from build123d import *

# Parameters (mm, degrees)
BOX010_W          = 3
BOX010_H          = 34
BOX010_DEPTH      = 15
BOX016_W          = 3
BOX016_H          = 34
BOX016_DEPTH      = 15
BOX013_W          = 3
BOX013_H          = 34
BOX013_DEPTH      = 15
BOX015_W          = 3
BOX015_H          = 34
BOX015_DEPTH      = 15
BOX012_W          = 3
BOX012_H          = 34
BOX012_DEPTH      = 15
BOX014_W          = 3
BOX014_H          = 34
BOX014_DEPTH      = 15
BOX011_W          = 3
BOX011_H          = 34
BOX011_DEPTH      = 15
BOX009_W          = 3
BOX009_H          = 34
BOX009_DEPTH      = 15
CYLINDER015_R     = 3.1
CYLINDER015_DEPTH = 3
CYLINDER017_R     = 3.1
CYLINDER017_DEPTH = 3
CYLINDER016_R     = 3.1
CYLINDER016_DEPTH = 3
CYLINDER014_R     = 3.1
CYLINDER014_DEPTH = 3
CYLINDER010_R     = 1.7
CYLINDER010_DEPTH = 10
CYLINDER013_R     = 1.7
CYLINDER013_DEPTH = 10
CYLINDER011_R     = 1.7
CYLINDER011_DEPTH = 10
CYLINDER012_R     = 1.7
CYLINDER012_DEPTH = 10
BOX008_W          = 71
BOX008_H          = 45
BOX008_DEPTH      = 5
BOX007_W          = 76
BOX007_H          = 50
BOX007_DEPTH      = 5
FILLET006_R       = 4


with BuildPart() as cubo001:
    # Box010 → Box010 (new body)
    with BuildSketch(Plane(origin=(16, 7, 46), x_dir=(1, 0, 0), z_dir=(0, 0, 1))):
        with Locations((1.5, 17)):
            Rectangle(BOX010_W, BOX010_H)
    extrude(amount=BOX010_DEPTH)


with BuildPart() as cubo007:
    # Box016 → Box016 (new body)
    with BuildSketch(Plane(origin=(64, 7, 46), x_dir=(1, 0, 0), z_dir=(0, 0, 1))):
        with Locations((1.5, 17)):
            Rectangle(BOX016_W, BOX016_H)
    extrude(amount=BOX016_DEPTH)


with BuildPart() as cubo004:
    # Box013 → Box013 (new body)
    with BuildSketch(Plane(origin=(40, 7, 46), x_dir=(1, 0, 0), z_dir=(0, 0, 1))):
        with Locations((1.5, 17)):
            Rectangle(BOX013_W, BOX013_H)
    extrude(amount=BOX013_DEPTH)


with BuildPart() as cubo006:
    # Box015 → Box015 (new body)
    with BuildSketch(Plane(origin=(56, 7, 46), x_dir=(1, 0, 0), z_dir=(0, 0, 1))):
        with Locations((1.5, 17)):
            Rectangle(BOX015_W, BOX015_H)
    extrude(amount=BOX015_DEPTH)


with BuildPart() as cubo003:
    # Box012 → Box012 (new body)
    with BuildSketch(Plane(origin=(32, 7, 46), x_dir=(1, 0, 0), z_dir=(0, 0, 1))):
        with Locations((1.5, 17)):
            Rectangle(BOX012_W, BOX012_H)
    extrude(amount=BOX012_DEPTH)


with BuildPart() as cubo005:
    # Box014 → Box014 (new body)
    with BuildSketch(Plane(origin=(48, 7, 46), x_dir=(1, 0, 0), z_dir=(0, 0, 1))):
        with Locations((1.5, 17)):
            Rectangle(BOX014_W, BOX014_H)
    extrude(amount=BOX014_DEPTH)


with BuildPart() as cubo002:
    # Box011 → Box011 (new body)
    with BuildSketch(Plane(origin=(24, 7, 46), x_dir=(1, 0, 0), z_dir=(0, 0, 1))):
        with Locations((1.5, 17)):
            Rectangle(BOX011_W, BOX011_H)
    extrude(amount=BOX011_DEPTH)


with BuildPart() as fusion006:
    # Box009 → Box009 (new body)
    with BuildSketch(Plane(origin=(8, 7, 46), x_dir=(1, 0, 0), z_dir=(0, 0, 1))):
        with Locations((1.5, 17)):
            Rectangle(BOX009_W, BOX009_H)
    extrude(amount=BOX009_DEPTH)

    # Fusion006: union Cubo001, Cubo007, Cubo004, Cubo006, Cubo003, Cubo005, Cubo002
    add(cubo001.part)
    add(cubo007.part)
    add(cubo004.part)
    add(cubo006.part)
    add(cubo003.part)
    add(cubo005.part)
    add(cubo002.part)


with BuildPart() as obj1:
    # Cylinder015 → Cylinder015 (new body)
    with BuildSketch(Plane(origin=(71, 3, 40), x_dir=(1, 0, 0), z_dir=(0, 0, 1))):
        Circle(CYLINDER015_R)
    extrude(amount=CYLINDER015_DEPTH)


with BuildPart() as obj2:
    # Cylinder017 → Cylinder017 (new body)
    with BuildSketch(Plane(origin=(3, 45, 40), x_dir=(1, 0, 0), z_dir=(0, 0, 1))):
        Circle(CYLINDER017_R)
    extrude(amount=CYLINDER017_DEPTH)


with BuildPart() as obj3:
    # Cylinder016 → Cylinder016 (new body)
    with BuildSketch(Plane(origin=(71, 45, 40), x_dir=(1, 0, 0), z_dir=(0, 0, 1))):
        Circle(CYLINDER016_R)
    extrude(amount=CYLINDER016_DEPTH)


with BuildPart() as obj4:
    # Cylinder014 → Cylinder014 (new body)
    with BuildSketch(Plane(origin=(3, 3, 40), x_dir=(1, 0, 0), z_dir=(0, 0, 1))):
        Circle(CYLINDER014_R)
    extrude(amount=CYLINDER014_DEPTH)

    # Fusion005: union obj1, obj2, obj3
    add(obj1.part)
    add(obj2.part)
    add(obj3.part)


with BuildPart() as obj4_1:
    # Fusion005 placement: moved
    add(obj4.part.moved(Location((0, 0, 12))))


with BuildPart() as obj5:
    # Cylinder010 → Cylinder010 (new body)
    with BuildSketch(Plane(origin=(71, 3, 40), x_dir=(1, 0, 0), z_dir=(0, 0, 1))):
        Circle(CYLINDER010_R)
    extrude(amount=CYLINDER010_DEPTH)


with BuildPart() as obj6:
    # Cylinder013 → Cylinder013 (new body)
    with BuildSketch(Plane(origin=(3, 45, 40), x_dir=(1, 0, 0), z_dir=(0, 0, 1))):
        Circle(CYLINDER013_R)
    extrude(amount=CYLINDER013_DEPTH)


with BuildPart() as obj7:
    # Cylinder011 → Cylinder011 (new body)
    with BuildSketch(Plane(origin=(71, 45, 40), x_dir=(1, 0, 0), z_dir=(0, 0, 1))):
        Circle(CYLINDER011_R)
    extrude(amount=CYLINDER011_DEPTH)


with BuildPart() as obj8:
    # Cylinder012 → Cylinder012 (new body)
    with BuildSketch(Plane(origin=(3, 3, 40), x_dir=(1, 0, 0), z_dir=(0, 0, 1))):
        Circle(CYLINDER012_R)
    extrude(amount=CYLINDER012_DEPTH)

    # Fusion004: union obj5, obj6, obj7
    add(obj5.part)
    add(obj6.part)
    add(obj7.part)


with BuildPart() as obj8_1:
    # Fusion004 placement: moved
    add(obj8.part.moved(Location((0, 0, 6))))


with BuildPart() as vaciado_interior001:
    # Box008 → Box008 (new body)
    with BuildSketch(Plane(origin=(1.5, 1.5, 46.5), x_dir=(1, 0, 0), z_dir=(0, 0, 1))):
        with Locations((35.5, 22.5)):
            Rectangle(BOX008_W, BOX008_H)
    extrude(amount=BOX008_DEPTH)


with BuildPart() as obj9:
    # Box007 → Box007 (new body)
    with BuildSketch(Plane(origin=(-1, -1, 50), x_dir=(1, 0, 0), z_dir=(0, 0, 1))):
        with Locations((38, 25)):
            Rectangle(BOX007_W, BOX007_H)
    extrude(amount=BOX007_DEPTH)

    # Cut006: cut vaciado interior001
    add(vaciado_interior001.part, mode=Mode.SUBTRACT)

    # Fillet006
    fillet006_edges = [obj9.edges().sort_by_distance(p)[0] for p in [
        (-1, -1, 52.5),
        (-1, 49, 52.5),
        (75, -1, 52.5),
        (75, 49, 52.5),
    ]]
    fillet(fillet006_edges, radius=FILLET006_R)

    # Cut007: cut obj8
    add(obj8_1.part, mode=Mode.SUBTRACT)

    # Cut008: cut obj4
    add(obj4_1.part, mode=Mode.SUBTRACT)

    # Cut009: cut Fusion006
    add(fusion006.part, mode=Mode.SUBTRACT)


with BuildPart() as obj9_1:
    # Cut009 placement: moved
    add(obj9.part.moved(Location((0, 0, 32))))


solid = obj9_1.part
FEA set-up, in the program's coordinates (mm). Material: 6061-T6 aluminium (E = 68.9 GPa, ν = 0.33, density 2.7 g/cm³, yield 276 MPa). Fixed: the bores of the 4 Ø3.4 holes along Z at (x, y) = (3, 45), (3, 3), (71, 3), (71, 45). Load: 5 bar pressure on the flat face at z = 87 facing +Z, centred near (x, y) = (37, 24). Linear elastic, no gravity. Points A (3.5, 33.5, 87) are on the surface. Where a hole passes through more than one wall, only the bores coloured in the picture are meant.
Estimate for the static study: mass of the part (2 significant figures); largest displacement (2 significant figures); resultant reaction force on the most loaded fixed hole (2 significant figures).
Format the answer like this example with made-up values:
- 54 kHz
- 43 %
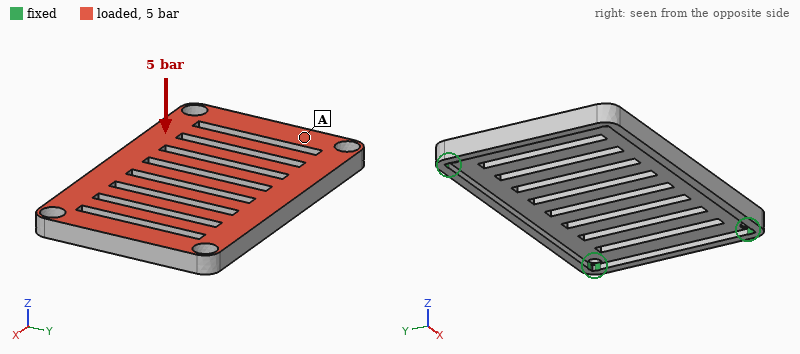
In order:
- 29 g
- 0.34 mm
- 810 N
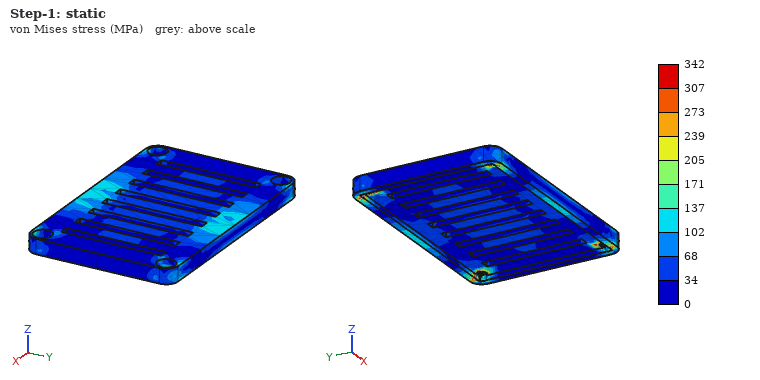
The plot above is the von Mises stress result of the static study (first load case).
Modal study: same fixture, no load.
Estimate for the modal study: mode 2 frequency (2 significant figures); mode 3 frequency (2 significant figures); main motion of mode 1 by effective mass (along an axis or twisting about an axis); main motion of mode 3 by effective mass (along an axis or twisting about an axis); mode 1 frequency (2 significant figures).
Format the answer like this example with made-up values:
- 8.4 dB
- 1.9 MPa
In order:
- 4000 Hz
- 5100 Hz
- along Z
- twisting about Y
- 2400 Hz
